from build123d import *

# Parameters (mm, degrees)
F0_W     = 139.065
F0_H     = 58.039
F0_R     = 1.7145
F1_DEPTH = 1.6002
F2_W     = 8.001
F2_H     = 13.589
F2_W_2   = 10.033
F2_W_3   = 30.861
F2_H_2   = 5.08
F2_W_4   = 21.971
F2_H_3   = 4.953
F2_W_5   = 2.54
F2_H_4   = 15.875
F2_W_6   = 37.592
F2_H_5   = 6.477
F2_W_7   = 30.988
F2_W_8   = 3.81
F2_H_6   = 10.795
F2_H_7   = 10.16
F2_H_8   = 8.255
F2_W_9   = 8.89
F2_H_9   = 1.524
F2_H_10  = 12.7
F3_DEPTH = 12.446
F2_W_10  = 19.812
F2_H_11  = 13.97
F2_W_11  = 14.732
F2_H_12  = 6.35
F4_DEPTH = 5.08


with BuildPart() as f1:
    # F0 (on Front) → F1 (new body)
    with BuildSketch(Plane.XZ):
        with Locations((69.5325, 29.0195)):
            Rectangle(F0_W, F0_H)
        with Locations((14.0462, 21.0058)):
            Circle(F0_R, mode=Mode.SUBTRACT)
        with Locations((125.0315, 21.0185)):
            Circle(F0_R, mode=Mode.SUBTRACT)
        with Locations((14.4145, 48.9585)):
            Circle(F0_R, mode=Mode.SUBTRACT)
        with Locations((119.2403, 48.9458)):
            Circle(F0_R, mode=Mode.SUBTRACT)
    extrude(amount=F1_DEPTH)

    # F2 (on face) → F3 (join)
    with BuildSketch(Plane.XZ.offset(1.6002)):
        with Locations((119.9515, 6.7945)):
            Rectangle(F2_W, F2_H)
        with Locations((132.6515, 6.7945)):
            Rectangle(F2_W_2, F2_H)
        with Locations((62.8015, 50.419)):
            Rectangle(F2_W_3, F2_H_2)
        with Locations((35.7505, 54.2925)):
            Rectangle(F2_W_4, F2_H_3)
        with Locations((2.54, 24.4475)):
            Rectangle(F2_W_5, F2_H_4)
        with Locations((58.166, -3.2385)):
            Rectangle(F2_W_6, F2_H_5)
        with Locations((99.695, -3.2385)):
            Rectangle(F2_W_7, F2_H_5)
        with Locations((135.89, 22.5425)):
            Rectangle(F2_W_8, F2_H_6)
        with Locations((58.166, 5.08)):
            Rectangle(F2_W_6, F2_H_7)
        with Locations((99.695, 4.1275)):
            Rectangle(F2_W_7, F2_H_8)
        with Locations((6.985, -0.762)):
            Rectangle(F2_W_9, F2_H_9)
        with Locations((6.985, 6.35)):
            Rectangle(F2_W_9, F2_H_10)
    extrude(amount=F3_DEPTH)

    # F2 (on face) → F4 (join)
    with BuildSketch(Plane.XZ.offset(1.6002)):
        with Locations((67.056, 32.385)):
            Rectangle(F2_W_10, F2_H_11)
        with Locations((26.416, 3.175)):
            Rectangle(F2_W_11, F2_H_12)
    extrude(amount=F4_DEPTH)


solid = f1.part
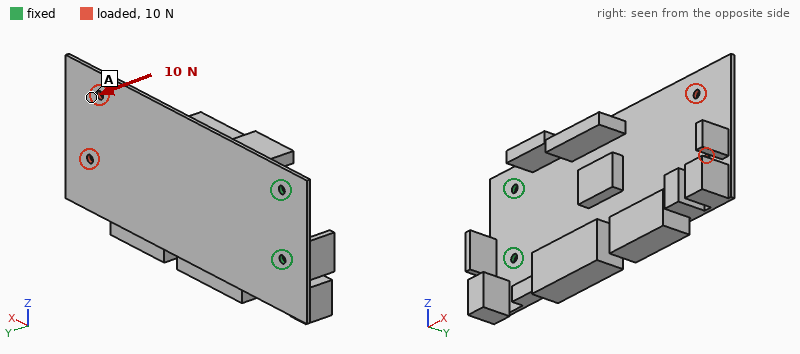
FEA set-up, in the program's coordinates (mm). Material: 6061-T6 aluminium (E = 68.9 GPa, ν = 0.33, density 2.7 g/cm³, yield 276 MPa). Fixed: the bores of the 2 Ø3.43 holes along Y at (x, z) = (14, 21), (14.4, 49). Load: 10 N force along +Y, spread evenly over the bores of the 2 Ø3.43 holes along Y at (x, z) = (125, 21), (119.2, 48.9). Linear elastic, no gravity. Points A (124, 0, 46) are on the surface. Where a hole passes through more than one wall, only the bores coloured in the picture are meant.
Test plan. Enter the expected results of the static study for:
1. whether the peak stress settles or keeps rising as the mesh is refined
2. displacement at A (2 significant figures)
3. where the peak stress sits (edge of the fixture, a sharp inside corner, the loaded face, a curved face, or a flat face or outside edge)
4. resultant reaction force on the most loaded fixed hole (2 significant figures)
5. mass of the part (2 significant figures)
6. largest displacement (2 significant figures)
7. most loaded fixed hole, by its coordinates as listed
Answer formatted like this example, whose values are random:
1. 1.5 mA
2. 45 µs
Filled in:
1. keeps rising
2. 1.5 mm
3. edge of the fixture
4. 10 N
5. 100 g
6. 1.7 mm
7. (14.4, 49)
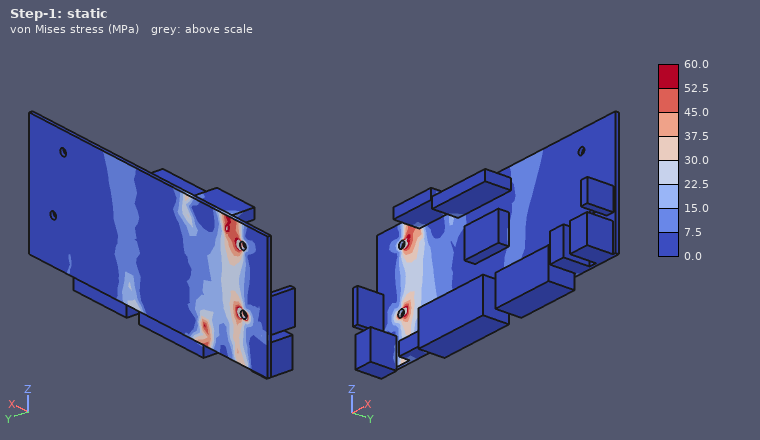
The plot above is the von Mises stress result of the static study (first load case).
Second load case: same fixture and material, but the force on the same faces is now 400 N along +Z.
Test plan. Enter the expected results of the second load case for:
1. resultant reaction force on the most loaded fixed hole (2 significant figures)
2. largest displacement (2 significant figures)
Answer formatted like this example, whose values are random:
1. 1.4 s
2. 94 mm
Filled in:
1. 1.5 kN
2. 0.19 mm
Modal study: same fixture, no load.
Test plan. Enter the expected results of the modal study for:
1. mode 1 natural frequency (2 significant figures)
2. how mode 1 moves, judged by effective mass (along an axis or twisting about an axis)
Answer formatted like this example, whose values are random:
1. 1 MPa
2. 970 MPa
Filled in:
1. 70 Hz
2. along Y
